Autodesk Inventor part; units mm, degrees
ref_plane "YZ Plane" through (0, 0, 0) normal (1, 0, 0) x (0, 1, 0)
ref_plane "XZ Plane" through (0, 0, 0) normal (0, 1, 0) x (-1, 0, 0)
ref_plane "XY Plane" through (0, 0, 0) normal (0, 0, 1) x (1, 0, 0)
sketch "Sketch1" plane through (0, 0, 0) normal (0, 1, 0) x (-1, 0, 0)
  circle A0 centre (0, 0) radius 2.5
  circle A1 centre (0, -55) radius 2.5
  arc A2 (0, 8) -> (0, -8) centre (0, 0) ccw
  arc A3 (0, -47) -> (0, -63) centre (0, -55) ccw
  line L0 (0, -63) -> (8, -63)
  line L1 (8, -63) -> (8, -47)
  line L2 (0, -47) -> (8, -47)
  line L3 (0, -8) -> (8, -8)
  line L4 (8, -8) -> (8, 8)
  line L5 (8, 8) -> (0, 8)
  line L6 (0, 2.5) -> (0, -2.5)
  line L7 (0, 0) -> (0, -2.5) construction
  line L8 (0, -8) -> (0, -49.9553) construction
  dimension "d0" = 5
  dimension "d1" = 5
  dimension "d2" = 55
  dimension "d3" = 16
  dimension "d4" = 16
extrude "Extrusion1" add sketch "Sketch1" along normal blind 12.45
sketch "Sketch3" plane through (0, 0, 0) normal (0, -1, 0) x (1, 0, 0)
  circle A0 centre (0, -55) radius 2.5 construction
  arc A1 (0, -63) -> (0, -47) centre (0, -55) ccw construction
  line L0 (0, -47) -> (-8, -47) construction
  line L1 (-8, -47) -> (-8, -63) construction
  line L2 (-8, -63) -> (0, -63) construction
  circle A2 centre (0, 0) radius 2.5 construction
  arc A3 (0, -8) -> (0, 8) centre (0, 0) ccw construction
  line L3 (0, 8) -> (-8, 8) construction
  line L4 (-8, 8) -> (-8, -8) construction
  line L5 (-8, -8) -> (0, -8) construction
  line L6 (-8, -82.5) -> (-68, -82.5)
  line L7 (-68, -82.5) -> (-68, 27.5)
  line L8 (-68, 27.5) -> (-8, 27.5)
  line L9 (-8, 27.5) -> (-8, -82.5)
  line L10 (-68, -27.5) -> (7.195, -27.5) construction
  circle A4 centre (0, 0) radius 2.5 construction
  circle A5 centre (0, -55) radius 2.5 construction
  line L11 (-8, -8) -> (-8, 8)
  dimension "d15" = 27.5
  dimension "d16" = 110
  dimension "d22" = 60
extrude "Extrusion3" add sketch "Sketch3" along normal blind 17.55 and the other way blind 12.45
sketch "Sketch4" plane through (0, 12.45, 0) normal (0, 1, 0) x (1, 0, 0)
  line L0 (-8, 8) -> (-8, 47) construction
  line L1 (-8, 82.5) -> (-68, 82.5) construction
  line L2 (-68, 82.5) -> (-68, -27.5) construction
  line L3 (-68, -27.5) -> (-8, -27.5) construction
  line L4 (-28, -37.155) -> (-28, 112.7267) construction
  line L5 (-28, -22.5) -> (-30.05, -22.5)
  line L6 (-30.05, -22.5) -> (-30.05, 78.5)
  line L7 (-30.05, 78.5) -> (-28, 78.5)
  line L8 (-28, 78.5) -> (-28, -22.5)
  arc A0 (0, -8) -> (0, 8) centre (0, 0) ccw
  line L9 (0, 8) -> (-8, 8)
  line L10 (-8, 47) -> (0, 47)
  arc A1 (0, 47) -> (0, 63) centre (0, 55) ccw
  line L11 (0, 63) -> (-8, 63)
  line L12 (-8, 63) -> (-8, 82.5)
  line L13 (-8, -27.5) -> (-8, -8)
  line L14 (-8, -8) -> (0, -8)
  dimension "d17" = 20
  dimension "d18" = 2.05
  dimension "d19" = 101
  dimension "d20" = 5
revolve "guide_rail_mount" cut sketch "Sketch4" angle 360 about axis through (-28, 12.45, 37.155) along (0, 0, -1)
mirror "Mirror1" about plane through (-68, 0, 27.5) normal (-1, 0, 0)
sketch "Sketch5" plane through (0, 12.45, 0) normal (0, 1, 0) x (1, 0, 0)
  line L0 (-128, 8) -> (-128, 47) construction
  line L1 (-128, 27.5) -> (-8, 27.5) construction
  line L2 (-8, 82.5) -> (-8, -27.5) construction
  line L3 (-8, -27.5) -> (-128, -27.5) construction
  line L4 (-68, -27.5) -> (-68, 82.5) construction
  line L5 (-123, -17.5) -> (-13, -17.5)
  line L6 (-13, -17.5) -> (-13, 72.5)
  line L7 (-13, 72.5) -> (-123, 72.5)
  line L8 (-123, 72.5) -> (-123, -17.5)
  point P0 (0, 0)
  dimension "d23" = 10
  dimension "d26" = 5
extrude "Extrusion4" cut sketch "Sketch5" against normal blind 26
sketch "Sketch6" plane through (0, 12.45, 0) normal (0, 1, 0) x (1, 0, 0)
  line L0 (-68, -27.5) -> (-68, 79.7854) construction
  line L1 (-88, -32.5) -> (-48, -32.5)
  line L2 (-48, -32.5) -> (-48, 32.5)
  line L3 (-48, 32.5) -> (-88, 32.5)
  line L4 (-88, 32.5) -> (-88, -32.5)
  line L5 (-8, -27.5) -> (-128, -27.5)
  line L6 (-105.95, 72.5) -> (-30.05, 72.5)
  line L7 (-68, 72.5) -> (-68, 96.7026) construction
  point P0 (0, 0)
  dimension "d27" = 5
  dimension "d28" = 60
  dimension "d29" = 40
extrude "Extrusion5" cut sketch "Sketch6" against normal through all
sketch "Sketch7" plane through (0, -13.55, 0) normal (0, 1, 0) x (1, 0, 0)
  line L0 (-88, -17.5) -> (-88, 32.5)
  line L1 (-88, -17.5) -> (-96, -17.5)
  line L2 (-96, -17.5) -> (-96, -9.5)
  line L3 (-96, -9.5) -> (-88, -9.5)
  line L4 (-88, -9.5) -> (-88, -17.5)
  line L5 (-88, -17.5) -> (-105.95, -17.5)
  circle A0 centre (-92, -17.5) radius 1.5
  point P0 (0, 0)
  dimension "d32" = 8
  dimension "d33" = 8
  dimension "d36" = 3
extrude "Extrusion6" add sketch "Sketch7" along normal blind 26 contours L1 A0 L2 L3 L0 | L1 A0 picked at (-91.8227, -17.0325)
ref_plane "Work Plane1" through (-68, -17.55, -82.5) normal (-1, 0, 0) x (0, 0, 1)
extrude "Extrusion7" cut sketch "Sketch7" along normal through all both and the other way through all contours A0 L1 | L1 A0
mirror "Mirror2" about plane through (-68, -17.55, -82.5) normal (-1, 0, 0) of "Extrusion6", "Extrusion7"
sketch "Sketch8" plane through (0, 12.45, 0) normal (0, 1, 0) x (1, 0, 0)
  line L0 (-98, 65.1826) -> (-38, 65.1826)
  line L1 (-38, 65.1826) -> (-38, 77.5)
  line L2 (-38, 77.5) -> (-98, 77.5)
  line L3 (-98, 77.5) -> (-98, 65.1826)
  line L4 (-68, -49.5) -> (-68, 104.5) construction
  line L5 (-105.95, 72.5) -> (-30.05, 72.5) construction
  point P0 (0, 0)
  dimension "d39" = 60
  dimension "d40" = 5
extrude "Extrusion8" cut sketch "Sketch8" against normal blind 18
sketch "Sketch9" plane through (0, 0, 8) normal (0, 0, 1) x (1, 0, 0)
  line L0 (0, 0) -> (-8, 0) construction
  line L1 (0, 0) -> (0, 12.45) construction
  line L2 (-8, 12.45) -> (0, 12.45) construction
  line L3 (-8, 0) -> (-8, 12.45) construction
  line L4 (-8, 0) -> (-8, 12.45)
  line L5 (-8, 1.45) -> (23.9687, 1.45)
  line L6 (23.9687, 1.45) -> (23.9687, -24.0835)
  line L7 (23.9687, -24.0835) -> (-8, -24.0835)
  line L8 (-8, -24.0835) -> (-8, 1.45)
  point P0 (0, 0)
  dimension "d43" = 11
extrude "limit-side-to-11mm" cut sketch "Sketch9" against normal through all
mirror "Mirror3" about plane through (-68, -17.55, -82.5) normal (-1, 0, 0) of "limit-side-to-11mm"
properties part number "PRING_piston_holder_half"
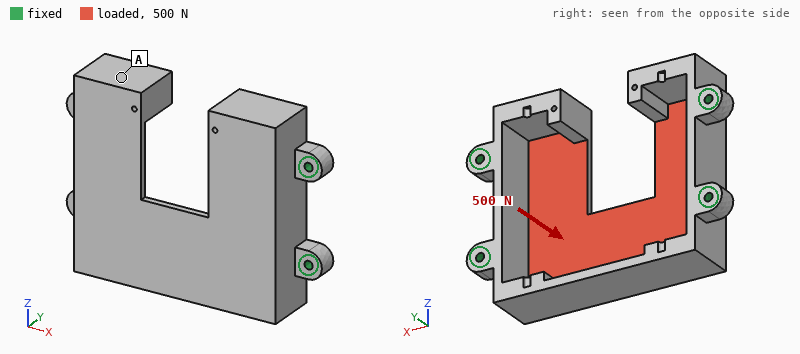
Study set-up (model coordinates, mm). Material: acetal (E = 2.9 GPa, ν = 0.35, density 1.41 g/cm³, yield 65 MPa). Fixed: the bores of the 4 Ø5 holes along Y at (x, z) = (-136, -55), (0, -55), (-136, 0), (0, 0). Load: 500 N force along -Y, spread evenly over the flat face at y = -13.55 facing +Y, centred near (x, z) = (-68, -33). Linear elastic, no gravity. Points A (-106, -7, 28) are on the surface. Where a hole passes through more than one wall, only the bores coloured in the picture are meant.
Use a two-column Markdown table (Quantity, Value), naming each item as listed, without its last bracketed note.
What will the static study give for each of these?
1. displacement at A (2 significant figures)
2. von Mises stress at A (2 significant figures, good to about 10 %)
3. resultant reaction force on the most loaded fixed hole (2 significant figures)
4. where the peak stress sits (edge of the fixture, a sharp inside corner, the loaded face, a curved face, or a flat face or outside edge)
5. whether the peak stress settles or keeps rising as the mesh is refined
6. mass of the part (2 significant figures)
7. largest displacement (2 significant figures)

| Quantity | Value |
|---|---|
| displacement at A | 0.17 mm |
| von Mises stress at A | 1.2 MPa |
| resultant reaction force on the most loaded fixed hole | 160 N |
| where the peak stress sits | a sharp inside corner |
| whether the peak stress settles or keeps rising as the mesh is refined | keeps rising |
| mass of the part | 180 g |
| largest displacement | 0.85 mm |
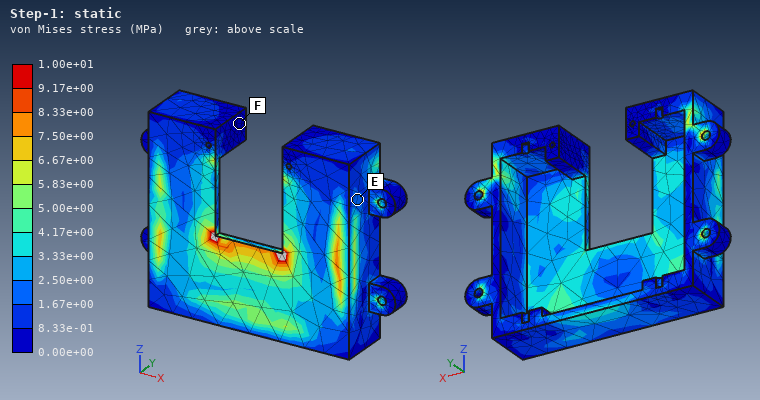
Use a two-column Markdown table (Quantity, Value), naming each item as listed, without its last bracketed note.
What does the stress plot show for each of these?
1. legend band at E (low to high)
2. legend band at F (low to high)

| Quantity | Value |
|---|---|
| legend band at E | 1.67e+00 to 2.50e+00 MPa |
| legend band at F | 0.00e+00 to 8.33e-01 MPa |
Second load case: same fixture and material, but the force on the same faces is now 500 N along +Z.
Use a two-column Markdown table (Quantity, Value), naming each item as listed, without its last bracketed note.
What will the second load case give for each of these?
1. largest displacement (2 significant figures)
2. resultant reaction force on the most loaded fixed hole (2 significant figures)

| Quantity | Value |
|---|---|
| largest displacement | 0.19 mm |
| resultant reaction force on the most loaded fixed hole | 160 N |
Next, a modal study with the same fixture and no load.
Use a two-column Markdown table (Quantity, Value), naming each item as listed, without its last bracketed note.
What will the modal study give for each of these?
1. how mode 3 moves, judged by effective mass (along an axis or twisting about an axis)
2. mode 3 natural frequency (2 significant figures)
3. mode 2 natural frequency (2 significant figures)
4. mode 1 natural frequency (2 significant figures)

| Quantity | Value |
|---|---|
| how mode 3 moves, judged by effective mass | along Y |
| mode 3 natural frequency | 840 Hz |
| mode 2 natural frequency | 550 Hz |
| mode 1 natural frequency | 530 Hz |
